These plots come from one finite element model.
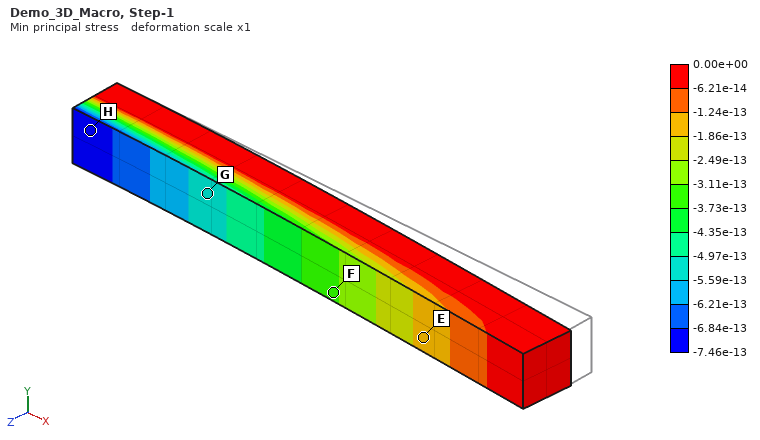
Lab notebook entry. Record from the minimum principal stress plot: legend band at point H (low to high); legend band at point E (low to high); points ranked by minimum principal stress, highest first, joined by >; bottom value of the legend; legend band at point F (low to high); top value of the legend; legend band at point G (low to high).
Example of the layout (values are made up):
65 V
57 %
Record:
-7.46e-13 to -6.84e-13
-1.86e-13 to -1.24e-13
E > F > G > H
-7.46e-13
-3.73e-13 to -3.11e-13
0.00e+00
-5.59e-13 to -4.97e-13
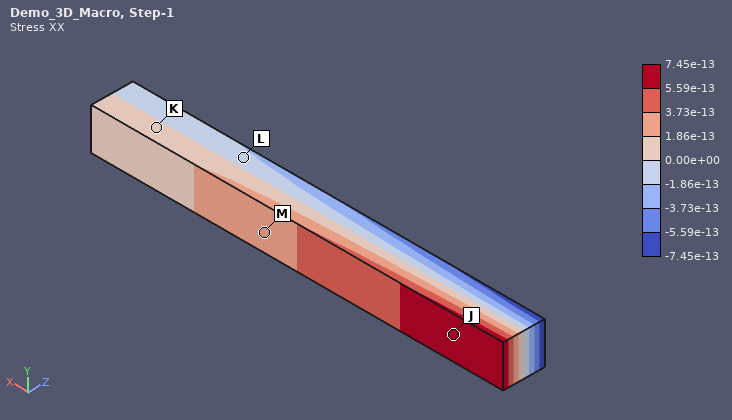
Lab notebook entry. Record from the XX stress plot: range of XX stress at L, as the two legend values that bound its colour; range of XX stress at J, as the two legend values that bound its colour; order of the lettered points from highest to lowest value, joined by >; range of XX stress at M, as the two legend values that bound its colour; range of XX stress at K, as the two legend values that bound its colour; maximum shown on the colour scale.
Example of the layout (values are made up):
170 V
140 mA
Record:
-1.86e-13 to 0.00e+00
5.59e-13 to 7.45e-13
J > M > K > L
1.86e-13 to 3.73e-13
0.00e+00 to 1.86e-13
7.45e-13
